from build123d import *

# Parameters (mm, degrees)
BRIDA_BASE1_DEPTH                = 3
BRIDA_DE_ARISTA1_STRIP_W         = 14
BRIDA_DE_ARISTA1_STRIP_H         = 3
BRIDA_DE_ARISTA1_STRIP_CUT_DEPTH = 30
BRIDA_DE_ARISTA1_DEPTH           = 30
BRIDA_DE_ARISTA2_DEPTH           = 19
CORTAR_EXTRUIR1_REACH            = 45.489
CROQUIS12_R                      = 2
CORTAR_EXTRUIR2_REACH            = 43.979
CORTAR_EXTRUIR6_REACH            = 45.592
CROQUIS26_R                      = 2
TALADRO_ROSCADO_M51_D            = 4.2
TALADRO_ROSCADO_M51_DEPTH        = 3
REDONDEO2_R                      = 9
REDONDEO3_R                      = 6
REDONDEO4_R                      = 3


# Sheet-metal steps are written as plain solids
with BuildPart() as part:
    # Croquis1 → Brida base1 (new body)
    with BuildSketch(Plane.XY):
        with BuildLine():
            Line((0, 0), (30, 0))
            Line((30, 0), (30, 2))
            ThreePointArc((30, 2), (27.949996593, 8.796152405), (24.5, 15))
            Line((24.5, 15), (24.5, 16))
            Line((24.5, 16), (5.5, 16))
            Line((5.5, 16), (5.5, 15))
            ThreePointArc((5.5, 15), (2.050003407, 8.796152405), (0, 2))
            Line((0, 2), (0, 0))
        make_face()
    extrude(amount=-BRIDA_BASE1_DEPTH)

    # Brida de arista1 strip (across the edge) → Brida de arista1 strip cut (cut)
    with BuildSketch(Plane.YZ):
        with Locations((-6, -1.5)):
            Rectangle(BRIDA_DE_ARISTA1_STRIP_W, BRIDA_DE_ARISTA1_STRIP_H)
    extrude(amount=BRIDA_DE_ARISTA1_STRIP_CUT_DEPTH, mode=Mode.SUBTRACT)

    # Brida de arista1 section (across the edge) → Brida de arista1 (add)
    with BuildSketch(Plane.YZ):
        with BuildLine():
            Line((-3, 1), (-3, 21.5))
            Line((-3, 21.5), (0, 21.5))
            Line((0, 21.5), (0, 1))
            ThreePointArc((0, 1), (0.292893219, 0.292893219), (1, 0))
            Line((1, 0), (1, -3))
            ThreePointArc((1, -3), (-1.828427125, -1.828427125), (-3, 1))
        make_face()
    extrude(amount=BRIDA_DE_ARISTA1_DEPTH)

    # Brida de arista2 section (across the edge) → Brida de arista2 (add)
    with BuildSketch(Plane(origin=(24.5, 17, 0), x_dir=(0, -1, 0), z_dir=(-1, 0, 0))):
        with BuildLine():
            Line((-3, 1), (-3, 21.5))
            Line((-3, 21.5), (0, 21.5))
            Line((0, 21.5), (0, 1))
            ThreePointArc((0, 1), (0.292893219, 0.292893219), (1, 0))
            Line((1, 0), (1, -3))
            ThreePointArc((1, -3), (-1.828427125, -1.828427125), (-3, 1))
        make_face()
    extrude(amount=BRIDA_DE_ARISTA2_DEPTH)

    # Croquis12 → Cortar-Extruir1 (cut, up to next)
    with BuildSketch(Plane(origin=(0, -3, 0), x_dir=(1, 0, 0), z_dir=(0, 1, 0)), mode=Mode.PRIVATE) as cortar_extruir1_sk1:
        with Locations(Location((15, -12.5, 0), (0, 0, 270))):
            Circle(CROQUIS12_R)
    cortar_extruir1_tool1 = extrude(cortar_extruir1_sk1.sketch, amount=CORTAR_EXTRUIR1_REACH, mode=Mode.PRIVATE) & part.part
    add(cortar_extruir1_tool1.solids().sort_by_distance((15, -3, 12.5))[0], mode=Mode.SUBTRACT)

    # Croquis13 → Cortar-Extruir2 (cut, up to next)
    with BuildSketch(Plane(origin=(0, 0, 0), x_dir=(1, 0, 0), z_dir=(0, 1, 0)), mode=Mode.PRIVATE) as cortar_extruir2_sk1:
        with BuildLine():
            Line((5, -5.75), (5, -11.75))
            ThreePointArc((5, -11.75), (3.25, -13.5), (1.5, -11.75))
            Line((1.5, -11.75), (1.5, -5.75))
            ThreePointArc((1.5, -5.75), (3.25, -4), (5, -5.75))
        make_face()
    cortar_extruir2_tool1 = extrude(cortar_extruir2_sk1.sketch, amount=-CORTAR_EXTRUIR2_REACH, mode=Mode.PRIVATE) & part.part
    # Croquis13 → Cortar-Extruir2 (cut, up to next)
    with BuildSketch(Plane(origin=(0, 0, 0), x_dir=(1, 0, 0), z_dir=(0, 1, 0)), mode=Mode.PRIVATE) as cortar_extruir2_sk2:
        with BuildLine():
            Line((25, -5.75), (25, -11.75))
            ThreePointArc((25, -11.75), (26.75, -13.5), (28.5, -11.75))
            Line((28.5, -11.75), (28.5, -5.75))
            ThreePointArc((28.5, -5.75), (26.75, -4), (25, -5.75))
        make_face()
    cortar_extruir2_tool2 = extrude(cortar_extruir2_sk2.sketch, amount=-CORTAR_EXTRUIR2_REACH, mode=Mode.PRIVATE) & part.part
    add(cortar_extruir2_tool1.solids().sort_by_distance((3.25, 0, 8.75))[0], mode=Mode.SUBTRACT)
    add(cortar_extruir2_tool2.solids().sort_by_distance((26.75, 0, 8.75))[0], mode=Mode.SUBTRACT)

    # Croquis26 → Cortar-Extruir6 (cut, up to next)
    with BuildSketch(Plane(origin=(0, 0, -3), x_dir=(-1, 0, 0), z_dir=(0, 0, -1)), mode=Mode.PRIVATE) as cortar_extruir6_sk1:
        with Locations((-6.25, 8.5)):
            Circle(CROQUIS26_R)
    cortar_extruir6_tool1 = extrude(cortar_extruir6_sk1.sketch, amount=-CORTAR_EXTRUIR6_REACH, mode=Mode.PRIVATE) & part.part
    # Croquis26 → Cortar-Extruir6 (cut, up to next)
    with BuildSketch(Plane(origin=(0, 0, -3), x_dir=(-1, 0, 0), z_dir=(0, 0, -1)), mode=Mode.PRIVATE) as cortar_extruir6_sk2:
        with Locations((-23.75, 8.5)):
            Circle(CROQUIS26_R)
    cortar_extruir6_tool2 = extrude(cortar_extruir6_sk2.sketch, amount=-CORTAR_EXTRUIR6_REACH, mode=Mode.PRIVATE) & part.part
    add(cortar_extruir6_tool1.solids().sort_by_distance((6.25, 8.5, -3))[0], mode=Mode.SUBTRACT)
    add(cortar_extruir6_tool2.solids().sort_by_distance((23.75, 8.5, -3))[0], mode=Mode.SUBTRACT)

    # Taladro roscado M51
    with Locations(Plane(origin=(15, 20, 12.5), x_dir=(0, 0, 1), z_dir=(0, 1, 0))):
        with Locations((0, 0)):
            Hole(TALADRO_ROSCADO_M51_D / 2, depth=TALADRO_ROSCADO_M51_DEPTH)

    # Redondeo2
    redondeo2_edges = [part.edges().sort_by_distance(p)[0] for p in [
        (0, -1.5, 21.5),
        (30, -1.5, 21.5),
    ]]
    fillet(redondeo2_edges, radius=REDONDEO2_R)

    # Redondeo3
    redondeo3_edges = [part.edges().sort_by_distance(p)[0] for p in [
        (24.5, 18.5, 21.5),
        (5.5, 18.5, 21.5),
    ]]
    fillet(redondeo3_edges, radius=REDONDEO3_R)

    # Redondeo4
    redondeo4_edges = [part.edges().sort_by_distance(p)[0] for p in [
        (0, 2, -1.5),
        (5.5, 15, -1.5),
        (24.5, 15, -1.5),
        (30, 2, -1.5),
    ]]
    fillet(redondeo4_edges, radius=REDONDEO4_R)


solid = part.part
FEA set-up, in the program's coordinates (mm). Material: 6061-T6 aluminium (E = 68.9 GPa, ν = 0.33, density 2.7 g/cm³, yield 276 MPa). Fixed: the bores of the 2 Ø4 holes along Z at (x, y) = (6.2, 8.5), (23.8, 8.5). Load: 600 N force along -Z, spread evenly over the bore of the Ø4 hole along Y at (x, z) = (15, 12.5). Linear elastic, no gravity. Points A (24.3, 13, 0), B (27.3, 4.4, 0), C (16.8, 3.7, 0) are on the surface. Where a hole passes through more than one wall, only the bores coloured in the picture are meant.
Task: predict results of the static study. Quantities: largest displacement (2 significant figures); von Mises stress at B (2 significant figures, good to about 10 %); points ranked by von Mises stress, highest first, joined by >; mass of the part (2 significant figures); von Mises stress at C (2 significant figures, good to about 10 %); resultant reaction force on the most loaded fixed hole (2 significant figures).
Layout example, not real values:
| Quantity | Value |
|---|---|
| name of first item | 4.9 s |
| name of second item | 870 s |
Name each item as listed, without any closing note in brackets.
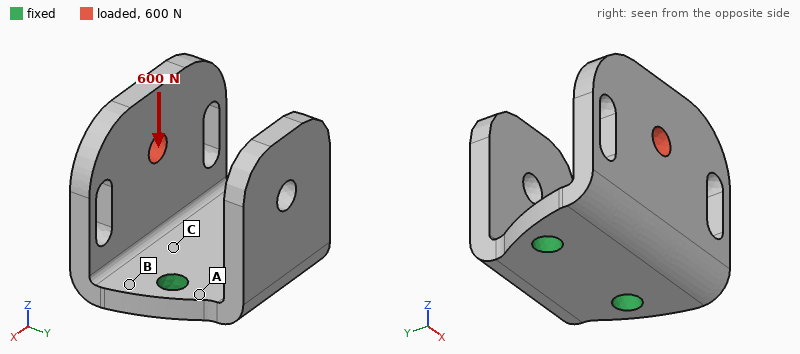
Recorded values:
| Quantity | Value |
|---|---|
| largest displacement | 0.14 mm |
| von Mises stress at B | 71 MPa |
| points ranked by von Mises stress, highest first, joined by > | B > C > A |
| mass of the part | 11 g |
| von Mises stress at C | 53 MPa |
| resultant reaction force on the most loaded fixed hole | 300 N |
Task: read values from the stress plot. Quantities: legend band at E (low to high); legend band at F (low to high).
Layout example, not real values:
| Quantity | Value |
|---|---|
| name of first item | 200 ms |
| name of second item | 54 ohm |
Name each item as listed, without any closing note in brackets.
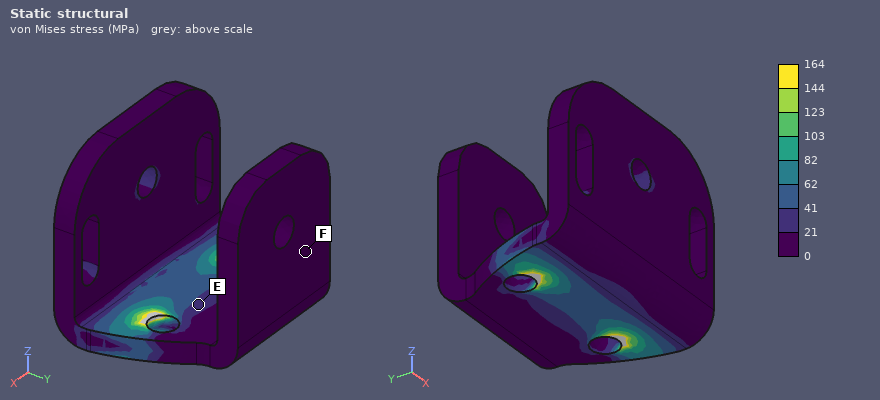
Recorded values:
| Quantity | Value |
|---|---|
| legend band at E | 21 to 41 MPa |
| legend band at F | 0 to 21 MPa |
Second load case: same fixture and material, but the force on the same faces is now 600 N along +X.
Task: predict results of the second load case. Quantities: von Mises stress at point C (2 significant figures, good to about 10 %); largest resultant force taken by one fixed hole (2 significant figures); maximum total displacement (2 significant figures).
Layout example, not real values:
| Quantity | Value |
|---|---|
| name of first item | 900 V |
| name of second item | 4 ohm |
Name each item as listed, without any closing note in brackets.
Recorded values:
| Quantity | Value |
|---|---|
| von Mises stress at point C | 63 MPa |
| largest resultant force taken by one fixed hole | 590 N |
| maximum total displacement | 95 µm |
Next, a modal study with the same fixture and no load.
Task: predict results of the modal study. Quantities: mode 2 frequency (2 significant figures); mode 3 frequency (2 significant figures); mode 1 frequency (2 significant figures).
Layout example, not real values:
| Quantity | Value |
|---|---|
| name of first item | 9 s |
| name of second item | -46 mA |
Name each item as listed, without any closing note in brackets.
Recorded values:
| Quantity | Value |
|---|---|
| mode 2 frequency | 3200 Hz |
| mode 3 frequency | 6700 Hz |
| mode 1 frequency | 3100 Hz |
